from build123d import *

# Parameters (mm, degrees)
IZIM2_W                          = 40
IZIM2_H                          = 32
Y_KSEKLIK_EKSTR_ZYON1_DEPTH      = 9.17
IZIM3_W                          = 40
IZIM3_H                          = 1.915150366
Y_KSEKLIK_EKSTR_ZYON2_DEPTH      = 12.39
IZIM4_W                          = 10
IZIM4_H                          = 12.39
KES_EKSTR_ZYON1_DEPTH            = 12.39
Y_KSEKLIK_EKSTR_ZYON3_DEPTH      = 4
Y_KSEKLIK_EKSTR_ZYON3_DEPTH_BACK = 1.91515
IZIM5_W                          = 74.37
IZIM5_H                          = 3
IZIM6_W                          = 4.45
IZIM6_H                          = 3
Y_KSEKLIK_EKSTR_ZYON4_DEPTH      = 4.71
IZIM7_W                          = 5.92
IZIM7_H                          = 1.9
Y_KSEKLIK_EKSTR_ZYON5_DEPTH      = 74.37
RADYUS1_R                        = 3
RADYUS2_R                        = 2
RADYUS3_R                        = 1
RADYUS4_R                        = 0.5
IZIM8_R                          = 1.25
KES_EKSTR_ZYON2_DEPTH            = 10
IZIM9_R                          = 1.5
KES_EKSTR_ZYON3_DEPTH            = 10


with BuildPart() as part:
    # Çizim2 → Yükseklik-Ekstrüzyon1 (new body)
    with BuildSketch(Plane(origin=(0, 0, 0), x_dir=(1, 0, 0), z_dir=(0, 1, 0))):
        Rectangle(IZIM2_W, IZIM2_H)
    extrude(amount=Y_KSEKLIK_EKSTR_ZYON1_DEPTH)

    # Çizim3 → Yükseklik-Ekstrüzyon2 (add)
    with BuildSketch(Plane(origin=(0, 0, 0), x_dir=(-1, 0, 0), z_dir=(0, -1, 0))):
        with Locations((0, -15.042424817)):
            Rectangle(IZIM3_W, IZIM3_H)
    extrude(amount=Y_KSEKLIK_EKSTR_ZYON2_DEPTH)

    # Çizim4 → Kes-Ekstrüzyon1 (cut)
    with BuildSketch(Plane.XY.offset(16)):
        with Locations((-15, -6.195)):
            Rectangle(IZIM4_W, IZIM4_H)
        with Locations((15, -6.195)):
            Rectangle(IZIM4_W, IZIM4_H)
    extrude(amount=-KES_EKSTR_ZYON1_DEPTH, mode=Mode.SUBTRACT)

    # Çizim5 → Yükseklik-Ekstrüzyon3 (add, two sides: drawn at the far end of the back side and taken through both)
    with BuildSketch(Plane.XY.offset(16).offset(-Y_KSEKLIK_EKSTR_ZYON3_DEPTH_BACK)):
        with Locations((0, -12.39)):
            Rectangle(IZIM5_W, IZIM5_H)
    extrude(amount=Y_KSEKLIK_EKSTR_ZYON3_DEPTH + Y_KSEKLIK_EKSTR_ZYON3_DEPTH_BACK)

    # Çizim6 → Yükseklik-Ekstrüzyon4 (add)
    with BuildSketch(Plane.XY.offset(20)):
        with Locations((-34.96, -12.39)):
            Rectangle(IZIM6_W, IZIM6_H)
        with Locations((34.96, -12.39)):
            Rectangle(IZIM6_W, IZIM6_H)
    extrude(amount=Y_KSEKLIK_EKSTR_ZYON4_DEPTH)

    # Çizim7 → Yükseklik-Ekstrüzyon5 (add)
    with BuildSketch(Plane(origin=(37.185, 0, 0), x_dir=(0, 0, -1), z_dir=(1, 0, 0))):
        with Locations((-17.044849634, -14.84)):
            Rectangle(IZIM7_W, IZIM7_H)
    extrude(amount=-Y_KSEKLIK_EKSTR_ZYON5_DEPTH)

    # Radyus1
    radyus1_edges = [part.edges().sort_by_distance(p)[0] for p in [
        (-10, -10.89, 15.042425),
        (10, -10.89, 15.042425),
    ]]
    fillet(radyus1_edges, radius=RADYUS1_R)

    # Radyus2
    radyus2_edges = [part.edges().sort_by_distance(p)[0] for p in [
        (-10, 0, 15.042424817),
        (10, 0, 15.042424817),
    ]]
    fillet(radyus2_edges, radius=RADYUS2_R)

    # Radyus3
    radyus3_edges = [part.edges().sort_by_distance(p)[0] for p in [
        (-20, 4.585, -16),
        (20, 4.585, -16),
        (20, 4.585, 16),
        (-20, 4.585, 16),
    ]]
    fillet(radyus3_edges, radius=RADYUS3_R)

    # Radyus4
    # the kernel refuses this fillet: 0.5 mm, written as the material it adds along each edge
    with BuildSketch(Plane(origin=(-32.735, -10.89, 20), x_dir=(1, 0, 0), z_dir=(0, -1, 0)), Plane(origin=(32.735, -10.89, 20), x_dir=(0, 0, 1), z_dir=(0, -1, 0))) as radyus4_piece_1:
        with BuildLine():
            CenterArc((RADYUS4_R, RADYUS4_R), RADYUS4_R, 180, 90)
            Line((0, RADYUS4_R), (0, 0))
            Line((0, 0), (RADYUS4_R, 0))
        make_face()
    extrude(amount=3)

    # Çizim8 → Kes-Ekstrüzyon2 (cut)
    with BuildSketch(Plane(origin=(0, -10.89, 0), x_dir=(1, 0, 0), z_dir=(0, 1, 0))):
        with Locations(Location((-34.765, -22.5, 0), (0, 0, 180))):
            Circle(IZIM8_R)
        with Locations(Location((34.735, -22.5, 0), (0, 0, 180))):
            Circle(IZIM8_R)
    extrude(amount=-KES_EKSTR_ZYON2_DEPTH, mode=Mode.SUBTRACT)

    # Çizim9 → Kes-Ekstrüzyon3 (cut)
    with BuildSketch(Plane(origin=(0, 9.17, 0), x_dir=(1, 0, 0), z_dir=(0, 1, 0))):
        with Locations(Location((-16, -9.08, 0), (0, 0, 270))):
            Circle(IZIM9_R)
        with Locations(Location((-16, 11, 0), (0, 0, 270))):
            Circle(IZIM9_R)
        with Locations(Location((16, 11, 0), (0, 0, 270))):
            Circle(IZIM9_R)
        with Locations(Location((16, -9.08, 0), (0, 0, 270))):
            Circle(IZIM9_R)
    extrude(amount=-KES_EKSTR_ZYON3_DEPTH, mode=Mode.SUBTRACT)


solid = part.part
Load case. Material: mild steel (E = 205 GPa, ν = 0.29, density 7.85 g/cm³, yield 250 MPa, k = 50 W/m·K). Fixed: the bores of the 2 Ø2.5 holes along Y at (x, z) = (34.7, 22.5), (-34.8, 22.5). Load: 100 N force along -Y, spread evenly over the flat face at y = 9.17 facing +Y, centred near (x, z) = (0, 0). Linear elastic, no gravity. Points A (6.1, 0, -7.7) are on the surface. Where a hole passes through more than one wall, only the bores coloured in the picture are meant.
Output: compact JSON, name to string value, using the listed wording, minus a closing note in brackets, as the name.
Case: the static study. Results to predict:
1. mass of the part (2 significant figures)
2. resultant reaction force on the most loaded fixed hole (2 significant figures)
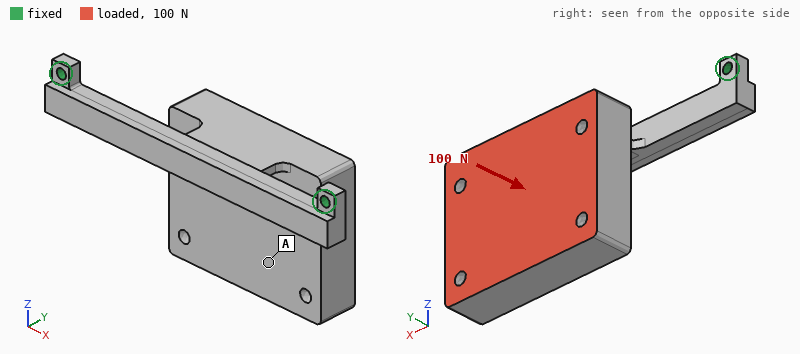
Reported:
{"mass of the part": "110 g", "resultant reaction force on the most loaded fixed hole": "57 N"}
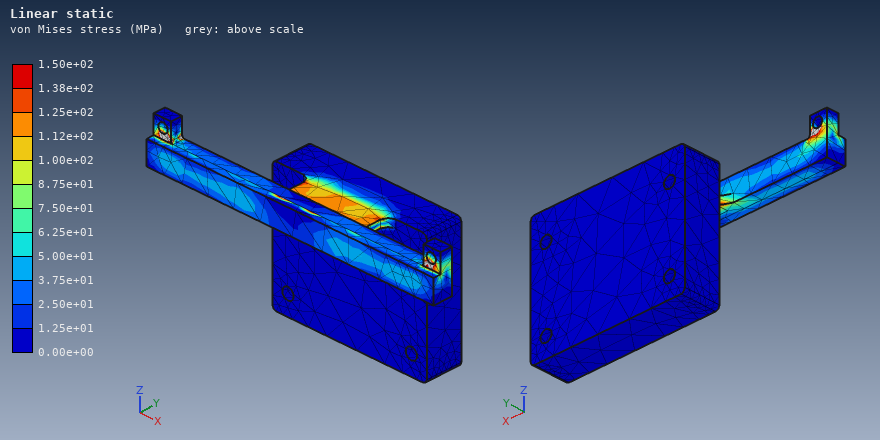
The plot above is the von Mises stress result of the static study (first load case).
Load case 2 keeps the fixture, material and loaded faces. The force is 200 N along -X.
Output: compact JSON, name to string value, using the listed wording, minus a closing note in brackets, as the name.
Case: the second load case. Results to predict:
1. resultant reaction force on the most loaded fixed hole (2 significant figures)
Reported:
{"resultant reaction force on the most loaded fixed hole": "140 N"}
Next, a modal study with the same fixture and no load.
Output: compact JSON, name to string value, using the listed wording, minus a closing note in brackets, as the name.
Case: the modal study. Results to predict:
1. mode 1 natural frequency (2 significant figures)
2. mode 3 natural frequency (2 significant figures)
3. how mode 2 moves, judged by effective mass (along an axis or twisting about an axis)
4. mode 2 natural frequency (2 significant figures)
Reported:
{"mode 1 natural frequency": "280 Hz", "mode 3 natural frequency": "1100 Hz", "how mode 2 moves, judged by effective mass": "along X", "mode 2 natural frequency": "650 Hz"}
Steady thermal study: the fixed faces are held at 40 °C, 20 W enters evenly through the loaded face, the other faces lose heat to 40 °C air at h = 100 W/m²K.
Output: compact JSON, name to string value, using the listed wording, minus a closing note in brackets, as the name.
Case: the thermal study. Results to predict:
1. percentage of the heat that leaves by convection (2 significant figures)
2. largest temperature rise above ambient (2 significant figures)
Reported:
{"percentage of the heat that leaves by convection": "93 %", "largest temperature rise above ambient": "56 K"}
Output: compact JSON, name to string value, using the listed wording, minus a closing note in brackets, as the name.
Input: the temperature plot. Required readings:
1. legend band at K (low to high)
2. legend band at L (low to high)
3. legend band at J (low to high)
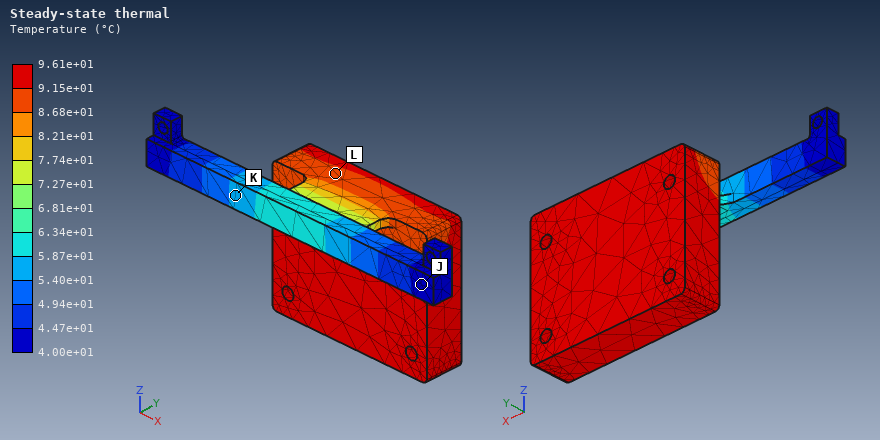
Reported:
{"legend band at K": "5.40e+01 to 5.87e+01 °C", "legend band at L": "8.68e+01 to 9.15e+01 °C", "legend band at J": "4.00e+01 to 4.47e+01 °C"}
